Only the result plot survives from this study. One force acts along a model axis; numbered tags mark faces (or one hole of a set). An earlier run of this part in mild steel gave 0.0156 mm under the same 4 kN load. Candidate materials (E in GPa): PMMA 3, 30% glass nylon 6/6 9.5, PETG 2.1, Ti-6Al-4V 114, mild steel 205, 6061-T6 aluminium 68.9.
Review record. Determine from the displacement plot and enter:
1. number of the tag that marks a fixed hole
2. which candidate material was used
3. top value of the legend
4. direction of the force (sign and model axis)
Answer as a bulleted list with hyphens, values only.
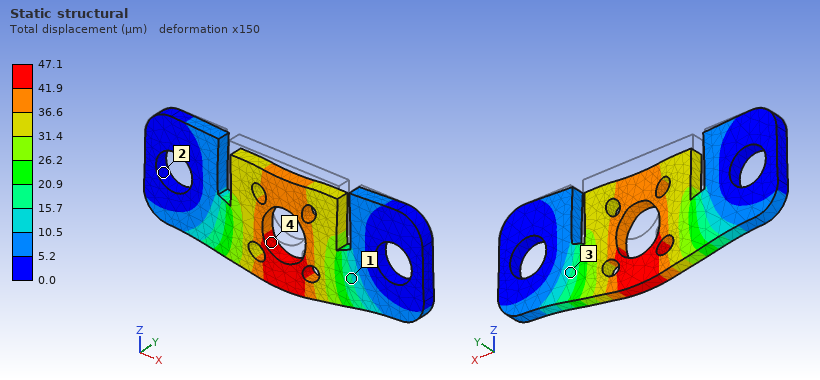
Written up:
- 2
- 6061-T6 aluminium
- 47.1 µm
- -Z
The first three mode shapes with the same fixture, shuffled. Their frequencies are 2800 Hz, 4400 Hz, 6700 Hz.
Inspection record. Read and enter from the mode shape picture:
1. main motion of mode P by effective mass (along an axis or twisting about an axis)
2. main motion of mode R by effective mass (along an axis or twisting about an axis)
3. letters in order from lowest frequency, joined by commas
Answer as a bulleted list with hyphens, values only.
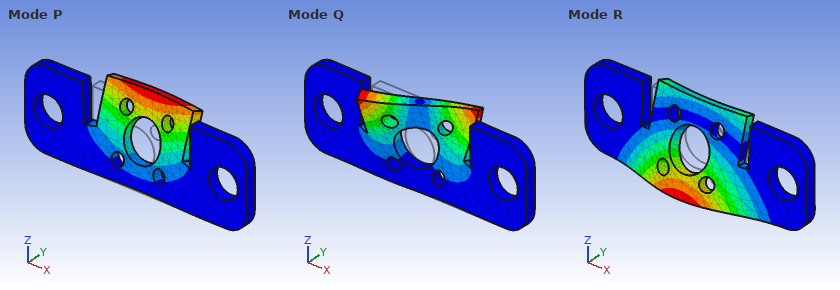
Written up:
- along Y
- along Y
- P, R, Q
